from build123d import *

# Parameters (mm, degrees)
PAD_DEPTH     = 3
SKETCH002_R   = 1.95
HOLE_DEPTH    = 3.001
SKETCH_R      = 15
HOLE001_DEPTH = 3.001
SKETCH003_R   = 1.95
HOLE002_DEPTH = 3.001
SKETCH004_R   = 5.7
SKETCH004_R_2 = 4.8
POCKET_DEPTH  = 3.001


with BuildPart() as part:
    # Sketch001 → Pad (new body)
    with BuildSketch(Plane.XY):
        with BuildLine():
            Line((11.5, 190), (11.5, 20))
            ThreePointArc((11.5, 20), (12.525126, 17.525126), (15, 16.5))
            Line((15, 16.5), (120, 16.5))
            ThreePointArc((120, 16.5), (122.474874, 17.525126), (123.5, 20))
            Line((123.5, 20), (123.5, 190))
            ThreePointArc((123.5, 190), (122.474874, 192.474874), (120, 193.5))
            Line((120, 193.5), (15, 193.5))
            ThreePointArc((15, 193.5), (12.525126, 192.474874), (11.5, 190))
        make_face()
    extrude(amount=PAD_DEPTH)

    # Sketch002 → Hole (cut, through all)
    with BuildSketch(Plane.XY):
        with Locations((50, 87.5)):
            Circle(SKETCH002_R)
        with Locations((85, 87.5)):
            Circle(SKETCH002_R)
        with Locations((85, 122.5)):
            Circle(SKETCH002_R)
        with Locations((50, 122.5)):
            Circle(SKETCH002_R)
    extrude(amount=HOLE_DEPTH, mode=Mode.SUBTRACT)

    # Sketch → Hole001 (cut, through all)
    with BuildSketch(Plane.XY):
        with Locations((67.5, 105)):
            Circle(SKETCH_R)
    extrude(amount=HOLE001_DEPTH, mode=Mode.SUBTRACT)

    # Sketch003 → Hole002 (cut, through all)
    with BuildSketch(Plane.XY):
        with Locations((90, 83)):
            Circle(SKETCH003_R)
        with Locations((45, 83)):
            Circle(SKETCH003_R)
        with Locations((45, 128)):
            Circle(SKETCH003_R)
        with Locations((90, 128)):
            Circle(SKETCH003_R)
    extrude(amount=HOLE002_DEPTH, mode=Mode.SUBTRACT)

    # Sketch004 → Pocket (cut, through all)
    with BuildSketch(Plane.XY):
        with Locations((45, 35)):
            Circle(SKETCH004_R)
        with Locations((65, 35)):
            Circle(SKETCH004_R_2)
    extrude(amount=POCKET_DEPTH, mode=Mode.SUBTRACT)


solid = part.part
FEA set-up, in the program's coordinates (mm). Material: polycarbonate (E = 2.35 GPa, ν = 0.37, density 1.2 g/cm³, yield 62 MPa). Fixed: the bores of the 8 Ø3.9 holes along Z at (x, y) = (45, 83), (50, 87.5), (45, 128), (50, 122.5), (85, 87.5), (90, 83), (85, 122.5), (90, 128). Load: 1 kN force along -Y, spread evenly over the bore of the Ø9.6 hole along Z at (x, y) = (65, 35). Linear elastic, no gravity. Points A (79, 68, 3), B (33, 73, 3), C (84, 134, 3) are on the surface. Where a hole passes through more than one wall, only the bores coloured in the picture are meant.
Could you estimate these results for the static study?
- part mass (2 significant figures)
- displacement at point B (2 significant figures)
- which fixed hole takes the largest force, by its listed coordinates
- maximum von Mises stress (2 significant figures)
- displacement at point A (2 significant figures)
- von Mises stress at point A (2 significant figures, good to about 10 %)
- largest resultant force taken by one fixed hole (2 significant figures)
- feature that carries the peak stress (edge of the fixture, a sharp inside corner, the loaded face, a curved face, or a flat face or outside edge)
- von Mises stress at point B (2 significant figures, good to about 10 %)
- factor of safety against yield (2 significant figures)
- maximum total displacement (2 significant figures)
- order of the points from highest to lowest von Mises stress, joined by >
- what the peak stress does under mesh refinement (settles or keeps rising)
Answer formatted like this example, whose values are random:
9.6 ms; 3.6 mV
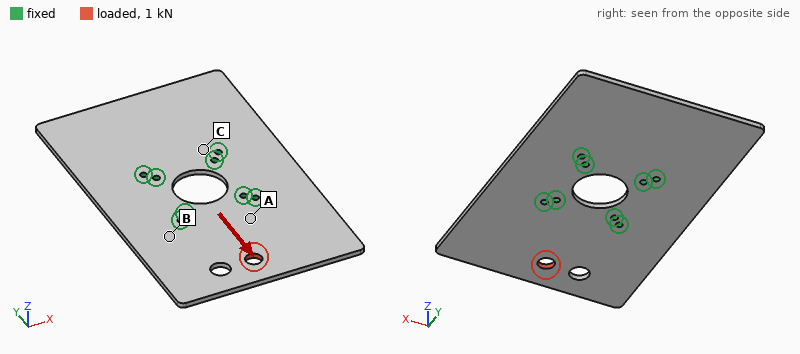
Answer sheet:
68 g; 0.041 mm; (45, 83); 24 MPa; 0.049 mm; 5.6 MPa; 290 N; the loaded face; 2.3 MPa; 2.6; 0.21 mm; A > B > C; settles
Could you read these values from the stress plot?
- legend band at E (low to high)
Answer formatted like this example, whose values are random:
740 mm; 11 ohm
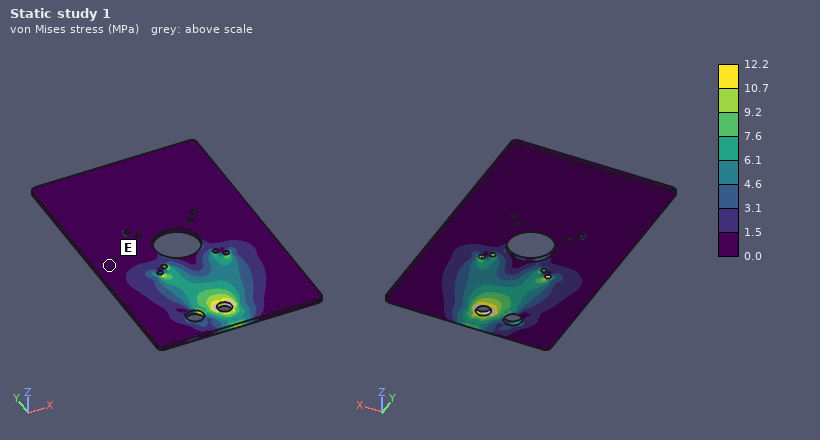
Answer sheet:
0.0 to 1.5 MPa
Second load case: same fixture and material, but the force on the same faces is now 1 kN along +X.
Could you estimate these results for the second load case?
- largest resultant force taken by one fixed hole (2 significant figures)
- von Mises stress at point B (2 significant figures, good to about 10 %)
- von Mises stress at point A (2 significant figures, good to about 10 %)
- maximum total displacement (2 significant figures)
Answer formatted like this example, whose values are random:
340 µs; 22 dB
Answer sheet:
610 N; 5.0 MPa; 9.1 MPa; 0.51 mm
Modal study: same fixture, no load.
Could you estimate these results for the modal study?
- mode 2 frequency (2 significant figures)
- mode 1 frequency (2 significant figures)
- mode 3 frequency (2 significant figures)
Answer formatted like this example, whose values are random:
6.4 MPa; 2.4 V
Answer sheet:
150 Hz; 150 Hz; 220 Hz
